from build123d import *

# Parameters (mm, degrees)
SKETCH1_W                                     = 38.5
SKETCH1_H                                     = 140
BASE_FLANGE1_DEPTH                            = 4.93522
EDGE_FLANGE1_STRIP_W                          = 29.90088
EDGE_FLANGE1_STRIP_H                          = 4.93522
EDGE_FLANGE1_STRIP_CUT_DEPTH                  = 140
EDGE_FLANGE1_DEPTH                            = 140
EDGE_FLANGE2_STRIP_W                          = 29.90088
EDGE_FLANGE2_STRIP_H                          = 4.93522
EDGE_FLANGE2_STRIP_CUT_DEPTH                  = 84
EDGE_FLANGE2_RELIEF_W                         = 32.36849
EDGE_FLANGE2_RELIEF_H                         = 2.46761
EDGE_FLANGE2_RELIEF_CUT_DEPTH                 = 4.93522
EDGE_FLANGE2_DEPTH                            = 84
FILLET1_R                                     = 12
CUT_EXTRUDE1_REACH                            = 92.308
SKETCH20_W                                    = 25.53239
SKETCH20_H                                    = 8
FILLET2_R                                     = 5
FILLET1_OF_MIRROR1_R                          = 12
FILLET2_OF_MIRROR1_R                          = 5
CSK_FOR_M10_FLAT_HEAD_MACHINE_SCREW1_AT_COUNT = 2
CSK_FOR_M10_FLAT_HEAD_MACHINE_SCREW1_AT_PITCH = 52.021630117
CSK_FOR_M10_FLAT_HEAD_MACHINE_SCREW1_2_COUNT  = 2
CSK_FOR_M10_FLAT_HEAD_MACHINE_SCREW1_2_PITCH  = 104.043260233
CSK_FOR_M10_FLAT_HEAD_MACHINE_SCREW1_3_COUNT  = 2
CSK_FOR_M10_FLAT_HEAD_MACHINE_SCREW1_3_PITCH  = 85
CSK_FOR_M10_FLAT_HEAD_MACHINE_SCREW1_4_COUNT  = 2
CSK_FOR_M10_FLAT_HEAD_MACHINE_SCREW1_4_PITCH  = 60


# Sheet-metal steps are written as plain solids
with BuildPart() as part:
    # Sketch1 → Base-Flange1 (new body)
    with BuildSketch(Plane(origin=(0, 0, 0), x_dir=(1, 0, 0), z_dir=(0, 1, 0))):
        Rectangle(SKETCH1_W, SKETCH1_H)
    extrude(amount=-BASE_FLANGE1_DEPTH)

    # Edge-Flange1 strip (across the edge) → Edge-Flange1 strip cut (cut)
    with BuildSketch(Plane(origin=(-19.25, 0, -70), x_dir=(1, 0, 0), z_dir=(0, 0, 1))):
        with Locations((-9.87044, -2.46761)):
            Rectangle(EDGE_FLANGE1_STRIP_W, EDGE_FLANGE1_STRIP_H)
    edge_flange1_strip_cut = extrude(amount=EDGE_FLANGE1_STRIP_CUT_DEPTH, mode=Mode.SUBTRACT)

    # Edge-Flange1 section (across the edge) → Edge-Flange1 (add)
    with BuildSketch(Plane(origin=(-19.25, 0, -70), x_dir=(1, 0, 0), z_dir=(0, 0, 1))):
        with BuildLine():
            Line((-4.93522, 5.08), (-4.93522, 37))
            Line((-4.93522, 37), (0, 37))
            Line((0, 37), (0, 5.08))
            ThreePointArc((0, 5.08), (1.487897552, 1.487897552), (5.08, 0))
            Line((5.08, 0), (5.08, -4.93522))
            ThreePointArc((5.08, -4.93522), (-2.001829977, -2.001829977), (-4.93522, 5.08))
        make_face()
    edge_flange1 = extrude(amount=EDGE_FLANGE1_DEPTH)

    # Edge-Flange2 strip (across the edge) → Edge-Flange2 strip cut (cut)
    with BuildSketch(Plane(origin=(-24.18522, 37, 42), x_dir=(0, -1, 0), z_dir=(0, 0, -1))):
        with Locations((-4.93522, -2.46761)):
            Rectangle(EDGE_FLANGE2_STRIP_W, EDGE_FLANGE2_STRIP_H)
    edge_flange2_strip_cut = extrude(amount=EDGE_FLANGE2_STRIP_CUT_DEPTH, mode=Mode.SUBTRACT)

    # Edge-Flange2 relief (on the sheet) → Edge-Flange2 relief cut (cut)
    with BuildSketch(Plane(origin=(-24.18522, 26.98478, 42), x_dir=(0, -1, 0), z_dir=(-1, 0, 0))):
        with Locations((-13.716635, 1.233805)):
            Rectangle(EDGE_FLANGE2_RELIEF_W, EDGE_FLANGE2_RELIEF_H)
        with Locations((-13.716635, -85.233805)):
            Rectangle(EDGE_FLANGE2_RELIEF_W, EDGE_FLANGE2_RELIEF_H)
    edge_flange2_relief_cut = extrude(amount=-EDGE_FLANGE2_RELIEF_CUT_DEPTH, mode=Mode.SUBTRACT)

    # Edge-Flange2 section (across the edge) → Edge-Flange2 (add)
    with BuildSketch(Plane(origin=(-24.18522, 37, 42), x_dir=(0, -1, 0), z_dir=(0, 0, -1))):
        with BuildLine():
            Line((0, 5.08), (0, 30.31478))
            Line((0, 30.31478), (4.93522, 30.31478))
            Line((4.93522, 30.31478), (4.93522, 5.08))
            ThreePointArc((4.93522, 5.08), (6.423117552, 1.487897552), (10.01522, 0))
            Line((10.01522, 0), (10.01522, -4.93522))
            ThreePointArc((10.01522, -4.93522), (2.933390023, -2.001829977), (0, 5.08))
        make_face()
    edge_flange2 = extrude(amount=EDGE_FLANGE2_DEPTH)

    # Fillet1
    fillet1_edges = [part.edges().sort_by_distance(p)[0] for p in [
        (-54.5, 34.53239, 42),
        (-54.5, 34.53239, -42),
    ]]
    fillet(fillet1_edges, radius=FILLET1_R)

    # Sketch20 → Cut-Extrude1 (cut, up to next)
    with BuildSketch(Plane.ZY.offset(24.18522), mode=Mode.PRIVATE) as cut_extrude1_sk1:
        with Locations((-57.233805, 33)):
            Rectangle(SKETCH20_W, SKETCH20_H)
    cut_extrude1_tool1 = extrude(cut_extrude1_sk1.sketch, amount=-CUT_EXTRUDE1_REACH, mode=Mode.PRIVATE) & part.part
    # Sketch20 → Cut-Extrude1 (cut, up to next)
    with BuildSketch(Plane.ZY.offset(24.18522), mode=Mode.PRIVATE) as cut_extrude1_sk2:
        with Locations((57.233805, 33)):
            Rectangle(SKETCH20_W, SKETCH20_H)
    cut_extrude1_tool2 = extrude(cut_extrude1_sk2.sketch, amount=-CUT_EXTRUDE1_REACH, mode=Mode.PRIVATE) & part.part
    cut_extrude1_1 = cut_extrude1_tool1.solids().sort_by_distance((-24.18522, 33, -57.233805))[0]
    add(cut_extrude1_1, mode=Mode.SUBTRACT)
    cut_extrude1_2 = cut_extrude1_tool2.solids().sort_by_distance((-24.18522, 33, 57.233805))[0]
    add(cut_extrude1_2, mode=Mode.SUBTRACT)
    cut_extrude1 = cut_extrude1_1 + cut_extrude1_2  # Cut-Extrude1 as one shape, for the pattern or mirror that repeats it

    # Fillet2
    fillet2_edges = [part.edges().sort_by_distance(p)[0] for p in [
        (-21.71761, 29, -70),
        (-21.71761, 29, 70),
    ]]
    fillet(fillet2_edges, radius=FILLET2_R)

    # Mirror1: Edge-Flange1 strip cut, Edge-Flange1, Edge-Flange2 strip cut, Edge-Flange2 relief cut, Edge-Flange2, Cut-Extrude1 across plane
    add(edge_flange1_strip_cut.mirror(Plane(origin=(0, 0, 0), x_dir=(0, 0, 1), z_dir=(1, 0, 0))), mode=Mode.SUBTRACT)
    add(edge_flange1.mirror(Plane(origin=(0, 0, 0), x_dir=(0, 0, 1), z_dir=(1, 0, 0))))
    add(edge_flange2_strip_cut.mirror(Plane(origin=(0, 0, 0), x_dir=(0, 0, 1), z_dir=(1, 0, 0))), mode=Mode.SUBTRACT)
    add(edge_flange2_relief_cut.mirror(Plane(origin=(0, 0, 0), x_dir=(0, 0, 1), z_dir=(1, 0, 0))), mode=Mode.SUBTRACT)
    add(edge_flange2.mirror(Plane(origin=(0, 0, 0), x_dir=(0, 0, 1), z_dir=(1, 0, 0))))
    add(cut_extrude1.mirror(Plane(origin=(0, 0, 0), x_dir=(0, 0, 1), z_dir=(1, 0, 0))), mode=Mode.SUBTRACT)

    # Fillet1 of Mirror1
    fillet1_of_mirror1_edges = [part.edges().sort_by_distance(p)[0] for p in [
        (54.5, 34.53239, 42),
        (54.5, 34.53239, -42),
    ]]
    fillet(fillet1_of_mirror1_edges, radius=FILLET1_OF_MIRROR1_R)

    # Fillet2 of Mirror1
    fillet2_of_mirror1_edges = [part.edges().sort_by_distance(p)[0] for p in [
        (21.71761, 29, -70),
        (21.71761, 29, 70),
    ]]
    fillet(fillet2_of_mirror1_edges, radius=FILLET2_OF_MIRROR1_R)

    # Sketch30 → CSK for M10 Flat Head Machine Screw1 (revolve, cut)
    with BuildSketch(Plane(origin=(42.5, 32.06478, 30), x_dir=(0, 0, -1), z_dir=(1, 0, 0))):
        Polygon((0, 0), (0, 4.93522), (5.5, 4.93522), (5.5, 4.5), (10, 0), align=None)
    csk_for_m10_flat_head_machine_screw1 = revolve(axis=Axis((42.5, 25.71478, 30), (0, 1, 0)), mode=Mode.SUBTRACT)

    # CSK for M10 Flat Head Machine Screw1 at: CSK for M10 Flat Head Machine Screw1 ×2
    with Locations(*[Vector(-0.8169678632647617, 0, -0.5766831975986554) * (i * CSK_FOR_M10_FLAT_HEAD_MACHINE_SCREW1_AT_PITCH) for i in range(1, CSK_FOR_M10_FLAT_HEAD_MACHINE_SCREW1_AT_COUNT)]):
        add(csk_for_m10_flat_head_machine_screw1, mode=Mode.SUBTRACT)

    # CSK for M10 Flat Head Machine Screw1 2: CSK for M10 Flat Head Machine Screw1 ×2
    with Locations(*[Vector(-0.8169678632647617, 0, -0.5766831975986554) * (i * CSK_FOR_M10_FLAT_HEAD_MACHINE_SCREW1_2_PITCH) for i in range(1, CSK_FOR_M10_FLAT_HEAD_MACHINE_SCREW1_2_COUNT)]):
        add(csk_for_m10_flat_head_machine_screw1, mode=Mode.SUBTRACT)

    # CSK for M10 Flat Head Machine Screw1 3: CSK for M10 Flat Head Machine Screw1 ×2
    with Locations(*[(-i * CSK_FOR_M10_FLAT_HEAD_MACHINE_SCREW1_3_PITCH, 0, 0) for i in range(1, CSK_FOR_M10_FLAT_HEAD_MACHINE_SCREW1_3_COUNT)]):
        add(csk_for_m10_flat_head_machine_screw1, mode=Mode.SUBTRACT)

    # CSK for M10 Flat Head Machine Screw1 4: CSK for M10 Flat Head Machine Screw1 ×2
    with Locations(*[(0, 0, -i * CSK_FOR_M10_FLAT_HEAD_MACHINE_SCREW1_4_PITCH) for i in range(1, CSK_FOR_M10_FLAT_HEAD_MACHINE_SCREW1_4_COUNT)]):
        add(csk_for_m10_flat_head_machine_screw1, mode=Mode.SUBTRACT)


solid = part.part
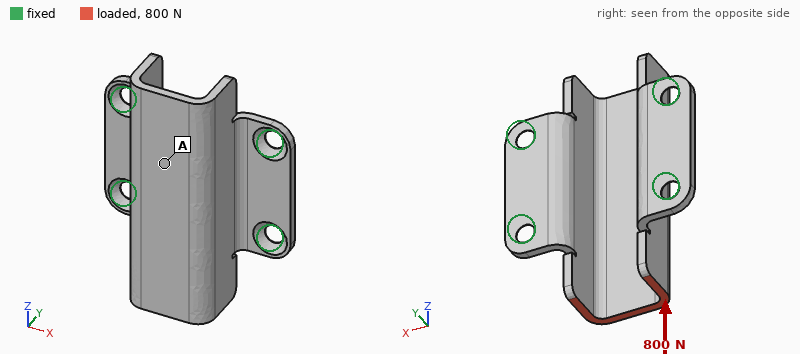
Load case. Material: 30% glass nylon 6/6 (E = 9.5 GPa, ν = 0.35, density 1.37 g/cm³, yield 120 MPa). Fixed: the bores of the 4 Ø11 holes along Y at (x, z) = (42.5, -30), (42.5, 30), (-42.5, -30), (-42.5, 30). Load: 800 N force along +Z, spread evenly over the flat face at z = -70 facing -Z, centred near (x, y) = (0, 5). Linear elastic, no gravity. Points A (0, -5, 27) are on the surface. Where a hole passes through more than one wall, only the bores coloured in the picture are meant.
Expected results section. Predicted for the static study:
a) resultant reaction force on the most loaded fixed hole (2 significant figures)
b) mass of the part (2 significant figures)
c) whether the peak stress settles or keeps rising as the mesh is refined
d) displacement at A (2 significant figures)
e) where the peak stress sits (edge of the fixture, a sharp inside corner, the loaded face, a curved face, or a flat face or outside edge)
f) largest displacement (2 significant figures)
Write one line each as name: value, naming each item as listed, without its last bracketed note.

resultant reaction force on the most loaded fixed hole: 360 N
mass of the part: 130 g
whether the peak stress settles or keeps rising as the mesh is refined: keeps rising
displacement at A: 0.16 mm
where the peak stress sits: edge of the fixture
largest displacement: 0.29 mm
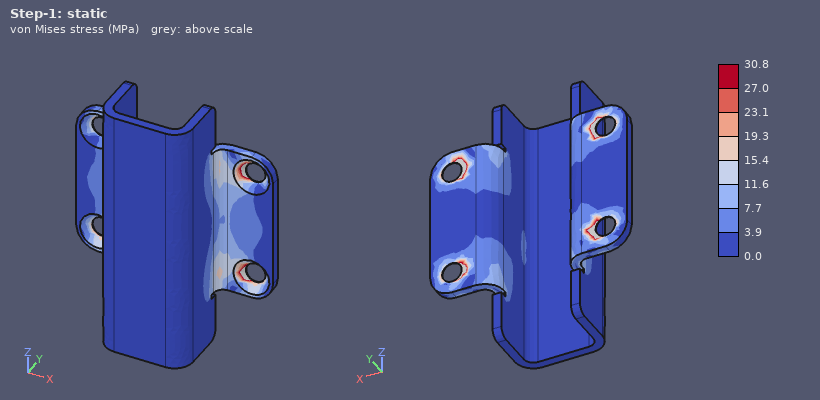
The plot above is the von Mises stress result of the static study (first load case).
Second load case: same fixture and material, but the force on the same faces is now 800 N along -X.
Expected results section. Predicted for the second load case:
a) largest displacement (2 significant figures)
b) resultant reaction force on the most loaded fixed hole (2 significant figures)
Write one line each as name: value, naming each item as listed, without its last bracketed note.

largest displacement: 1.2 mm
resultant reaction force on the most loaded fixed hole: 380 N
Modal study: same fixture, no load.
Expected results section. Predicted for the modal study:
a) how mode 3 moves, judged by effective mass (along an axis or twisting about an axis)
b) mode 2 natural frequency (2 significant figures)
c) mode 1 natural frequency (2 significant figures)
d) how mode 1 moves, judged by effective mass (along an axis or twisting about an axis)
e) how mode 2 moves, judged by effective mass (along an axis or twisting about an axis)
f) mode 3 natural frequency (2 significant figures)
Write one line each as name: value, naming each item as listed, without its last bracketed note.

how mode 3 moves, judged by effective mass: along X
mode 2 natural frequency: 950 Hz
mode 1 natural frequency: 840 Hz
how mode 1 moves, judged by effective mass: along Z
how mode 2 moves, judged by effective mass: twisting about Y
mode 3 natural frequency: 1100 Hz
